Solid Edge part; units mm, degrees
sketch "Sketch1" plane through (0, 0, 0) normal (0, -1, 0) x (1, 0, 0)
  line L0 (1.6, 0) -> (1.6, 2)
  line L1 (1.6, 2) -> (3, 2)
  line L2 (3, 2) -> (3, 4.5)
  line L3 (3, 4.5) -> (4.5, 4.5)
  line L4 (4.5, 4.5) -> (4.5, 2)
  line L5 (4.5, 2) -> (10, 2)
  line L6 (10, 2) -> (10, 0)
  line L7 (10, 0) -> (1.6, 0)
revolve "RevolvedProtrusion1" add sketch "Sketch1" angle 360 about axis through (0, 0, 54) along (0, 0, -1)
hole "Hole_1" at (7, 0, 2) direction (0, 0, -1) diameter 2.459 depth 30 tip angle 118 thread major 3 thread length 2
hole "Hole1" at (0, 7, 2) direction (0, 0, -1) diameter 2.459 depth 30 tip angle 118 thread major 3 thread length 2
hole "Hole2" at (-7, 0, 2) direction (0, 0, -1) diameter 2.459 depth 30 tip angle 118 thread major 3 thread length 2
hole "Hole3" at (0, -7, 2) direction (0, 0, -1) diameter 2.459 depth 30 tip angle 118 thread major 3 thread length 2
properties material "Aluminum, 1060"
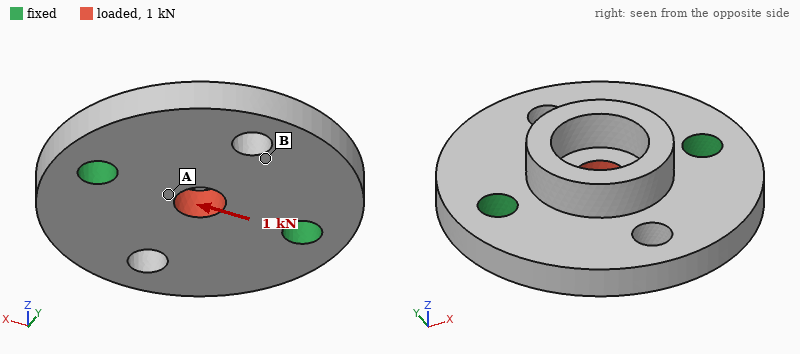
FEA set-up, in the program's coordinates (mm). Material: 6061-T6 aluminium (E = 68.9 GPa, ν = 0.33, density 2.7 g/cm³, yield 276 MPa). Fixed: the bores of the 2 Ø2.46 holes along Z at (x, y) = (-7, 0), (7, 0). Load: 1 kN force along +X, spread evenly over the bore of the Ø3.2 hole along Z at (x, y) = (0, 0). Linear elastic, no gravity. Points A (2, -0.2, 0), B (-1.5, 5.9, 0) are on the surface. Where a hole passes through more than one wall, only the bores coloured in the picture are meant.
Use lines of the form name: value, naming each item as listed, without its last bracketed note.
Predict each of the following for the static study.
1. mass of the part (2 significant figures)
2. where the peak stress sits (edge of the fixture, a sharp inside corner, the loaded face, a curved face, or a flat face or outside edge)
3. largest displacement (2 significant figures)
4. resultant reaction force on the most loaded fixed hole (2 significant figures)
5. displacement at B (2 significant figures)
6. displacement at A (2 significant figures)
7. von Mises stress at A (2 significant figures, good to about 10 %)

mass of the part: 1.8 g
where the peak stress sits: the loaded face
largest displacement: 3.8 µm
resultant reaction force on the most loaded fixed hole: 500 N
displacement at B: 1.7 µm
displacement at A: 3.0 µm
von Mises stress at A: 54 MPa
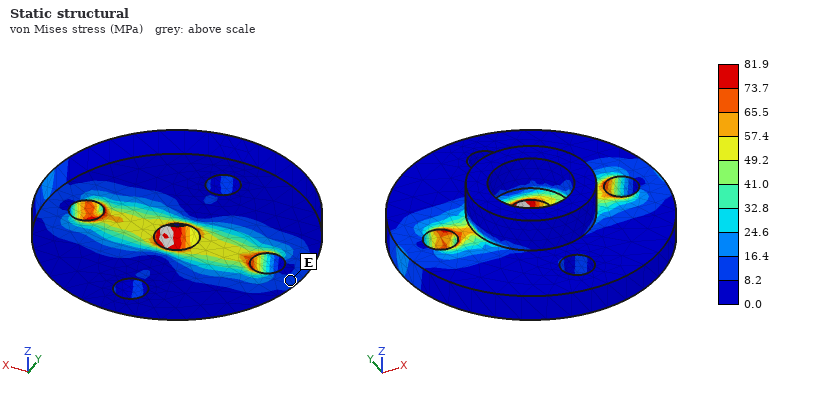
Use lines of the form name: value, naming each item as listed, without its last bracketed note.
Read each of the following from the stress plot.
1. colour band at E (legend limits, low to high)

colour band at E: 8.2 to 16.4 MPa
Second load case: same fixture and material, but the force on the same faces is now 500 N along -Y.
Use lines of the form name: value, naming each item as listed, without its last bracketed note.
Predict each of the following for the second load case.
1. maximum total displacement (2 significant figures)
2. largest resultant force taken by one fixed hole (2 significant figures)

maximum total displacement: 3.0 µm
largest resultant force taken by one fixed hole: 250 N
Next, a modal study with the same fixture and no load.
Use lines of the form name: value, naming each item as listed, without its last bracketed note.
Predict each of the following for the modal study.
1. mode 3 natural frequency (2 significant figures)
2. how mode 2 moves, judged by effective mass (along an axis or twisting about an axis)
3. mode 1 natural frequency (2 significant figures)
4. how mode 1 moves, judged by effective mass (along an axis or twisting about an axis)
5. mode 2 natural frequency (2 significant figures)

mode 3 natural frequency: 45 kHz
how mode 2 moves, judged by effective mass: along Z
mode 1 natural frequency: 19 kHz
how mode 1 moves, judged by effective mass: twisting about X
mode 2 natural frequency: 25 kHz
